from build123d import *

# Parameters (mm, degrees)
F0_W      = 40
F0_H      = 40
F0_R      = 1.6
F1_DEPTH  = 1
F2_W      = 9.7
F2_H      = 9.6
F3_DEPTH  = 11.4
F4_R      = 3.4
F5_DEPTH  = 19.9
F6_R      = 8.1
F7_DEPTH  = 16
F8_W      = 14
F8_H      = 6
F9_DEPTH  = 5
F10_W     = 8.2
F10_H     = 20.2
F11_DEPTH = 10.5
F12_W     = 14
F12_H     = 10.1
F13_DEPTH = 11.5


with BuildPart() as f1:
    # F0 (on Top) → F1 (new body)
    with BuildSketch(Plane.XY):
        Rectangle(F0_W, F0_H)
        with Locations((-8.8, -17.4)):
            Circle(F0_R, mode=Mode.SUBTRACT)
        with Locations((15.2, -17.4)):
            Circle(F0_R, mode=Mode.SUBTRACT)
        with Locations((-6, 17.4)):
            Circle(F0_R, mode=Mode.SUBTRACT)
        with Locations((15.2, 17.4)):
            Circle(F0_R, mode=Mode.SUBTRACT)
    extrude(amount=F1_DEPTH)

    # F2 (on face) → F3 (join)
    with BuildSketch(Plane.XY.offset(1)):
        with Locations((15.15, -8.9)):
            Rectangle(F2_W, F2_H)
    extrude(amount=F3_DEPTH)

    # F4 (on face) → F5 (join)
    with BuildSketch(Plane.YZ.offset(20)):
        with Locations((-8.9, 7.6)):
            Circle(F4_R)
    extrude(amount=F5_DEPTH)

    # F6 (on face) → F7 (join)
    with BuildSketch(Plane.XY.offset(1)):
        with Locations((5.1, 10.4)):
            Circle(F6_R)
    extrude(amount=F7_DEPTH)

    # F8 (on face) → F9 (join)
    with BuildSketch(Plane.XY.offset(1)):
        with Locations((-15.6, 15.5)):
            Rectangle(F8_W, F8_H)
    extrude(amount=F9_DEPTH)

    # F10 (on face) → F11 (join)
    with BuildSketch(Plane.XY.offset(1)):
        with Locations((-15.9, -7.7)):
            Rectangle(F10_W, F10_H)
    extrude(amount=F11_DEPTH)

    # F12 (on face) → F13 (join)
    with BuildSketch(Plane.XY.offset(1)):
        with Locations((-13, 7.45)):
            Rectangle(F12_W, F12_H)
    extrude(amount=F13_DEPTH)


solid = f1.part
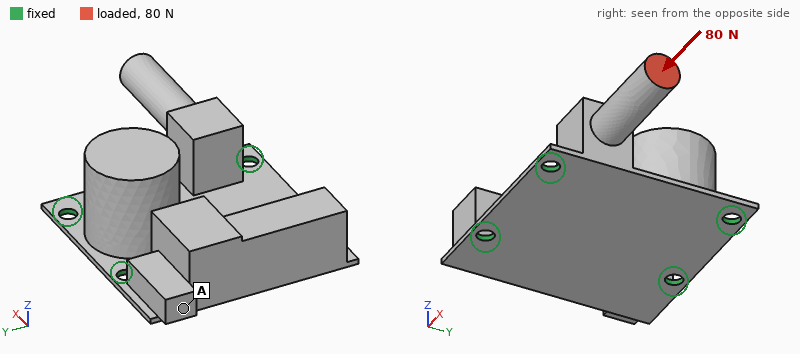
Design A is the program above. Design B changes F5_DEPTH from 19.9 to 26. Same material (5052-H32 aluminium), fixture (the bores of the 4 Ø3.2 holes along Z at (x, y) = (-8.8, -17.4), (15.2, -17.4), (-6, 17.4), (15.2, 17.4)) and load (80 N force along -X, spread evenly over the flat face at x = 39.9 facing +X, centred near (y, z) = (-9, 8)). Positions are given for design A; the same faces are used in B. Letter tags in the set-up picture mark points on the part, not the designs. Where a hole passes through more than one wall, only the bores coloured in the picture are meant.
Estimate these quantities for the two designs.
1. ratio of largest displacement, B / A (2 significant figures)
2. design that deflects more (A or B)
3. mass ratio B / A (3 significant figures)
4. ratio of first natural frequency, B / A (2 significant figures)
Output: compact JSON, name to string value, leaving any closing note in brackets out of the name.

{"ratio of largest displacement, B / A": "1.2", "design that deflects more": "B", "mass ratio B / A": "1.02", "ratio of first natural frequency, B / A": "0.90"}
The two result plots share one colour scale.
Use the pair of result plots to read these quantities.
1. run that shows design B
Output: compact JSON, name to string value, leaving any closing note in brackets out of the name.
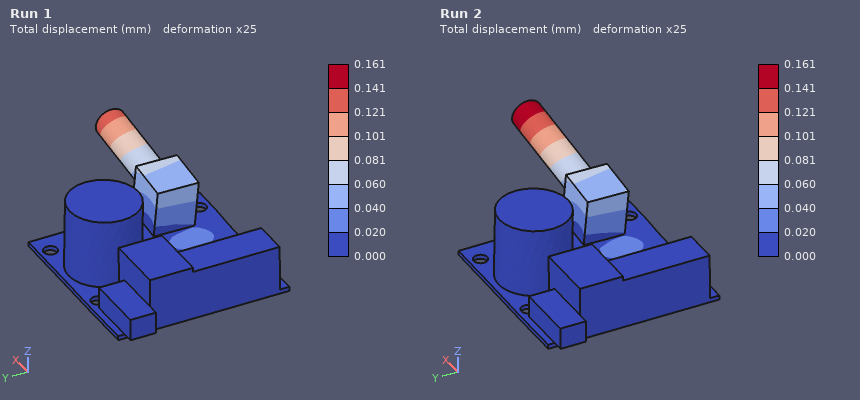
{"run that shows design B": "Run 2"}
